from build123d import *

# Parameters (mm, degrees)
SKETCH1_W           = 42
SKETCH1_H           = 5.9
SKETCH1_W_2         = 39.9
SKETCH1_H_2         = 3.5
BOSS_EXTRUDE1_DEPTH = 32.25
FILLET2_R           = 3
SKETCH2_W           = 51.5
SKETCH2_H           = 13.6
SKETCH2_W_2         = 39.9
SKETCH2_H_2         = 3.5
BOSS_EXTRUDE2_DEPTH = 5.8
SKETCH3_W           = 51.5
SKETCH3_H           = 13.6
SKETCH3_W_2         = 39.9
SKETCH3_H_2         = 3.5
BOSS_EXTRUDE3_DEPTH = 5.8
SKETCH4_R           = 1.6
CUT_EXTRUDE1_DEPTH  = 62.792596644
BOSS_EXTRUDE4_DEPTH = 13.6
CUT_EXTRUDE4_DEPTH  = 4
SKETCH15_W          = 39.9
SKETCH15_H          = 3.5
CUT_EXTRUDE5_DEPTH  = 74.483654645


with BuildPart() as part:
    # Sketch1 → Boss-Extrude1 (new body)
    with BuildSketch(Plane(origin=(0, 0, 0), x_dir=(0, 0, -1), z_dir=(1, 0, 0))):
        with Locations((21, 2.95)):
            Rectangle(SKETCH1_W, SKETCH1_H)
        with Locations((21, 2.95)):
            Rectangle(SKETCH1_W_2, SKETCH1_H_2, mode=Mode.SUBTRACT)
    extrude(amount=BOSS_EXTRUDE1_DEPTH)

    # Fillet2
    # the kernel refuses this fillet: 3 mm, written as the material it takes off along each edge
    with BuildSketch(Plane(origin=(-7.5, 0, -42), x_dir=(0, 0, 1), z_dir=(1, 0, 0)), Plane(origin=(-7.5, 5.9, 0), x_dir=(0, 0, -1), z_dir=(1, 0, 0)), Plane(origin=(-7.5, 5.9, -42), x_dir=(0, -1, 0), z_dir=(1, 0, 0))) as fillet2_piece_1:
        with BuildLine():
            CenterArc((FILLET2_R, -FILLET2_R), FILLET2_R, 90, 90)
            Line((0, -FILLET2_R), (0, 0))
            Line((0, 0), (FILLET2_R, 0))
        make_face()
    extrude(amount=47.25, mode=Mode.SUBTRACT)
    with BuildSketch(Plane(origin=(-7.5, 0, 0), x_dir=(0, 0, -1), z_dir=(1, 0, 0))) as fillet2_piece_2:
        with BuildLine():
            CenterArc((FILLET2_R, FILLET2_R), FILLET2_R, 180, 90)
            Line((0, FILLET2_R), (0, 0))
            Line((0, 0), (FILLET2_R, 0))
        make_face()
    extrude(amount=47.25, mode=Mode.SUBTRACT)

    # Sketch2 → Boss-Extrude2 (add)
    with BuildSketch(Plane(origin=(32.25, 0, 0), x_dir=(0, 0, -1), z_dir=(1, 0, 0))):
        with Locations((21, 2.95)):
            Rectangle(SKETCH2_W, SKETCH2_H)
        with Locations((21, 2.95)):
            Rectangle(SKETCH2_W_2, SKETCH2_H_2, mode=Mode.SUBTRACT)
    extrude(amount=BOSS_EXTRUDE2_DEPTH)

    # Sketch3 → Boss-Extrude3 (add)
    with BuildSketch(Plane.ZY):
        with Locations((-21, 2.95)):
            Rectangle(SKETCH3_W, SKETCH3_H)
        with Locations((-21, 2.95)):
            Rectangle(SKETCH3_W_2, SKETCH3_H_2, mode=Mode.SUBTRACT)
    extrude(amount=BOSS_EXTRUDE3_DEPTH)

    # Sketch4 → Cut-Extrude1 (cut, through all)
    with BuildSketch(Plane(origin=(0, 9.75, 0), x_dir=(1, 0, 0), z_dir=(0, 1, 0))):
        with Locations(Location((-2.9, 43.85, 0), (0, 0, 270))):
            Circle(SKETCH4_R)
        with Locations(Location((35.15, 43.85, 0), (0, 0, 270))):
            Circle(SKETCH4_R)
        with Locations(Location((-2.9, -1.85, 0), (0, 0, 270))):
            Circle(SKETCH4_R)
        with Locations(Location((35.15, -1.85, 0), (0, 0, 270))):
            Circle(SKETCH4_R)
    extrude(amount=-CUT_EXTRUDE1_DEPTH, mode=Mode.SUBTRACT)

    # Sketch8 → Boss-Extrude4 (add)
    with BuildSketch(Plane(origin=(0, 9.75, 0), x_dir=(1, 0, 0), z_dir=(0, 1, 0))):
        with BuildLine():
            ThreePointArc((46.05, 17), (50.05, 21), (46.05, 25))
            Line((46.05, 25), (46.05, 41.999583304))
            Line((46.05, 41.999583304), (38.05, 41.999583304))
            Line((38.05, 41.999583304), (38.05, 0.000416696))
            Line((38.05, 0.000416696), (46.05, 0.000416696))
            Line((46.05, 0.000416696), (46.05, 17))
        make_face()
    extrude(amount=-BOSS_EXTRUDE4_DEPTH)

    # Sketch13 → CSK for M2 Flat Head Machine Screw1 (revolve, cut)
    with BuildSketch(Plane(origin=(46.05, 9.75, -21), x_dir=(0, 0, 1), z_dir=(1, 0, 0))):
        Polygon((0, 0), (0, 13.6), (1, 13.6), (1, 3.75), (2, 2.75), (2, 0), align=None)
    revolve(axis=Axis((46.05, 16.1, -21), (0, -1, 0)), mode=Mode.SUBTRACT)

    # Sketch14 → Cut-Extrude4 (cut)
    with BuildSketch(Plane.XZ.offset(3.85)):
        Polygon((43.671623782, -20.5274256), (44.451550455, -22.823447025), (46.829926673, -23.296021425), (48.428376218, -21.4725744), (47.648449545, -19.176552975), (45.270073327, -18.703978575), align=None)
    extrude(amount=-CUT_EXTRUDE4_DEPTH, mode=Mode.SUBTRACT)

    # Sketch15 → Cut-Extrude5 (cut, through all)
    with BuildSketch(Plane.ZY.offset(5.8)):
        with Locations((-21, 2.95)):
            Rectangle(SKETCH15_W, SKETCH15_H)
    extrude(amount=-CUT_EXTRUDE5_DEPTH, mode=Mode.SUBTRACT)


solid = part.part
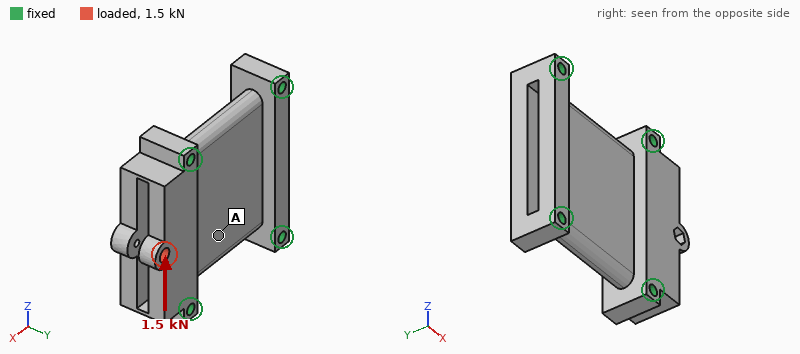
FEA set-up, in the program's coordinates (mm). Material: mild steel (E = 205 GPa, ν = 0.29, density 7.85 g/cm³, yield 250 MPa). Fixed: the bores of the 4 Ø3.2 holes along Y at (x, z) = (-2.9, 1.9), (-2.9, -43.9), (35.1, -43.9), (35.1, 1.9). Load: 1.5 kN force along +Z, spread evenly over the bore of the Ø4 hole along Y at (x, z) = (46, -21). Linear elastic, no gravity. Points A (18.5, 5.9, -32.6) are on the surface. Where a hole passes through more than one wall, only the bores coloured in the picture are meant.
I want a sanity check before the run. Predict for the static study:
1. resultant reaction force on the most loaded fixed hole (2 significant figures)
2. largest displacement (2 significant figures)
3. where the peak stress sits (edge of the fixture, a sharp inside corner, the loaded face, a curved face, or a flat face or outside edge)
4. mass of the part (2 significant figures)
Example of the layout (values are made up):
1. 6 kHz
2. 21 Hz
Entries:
1. 830 N
2. 6.3 µm
3. a flat face or outside edge
4. 100 g
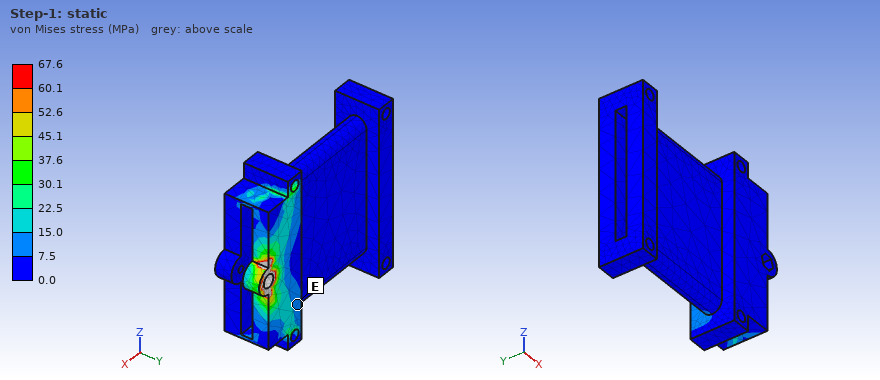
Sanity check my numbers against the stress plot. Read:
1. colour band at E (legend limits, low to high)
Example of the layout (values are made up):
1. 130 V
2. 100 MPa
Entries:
1. 7.5 to 15.0 MPa
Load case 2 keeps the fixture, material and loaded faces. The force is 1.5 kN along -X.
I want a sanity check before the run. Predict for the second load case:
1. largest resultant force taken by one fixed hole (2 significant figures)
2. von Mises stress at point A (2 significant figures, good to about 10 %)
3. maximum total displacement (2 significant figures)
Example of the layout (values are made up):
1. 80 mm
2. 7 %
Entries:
1. 690 N
2. 13 MPa
3. 15 µm
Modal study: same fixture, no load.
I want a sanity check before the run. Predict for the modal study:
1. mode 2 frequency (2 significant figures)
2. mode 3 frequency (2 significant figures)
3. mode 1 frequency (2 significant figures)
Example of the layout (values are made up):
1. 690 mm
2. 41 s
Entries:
1. 6500 Hz
2. 10 kHz
3. 6400 Hz
